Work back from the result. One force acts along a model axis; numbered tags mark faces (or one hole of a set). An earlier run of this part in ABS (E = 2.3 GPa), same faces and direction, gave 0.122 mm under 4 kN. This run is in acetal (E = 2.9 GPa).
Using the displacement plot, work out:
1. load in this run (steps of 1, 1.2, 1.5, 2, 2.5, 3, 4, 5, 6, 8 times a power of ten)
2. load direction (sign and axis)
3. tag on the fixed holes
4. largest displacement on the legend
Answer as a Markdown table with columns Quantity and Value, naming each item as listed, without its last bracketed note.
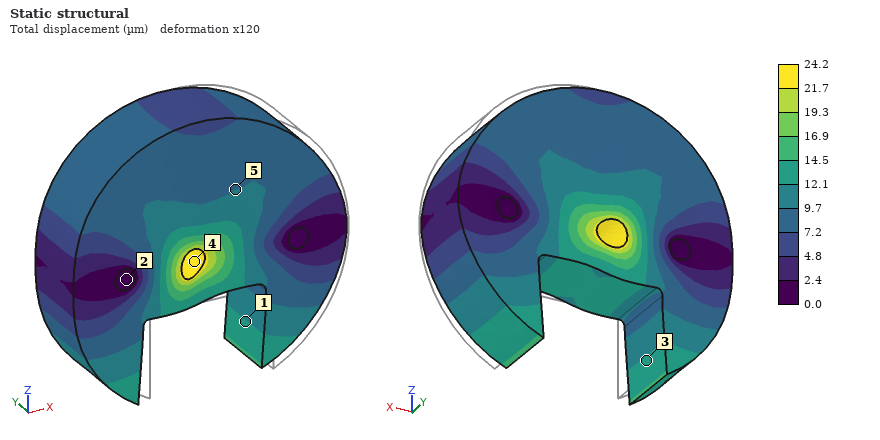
| Quantity | Value |
|---|---|
| load in this run | 1 kN |
| load direction | -X |
| tag on the fixed holes | 2 |
| largest displacement on the legend | 24.2 µm |
